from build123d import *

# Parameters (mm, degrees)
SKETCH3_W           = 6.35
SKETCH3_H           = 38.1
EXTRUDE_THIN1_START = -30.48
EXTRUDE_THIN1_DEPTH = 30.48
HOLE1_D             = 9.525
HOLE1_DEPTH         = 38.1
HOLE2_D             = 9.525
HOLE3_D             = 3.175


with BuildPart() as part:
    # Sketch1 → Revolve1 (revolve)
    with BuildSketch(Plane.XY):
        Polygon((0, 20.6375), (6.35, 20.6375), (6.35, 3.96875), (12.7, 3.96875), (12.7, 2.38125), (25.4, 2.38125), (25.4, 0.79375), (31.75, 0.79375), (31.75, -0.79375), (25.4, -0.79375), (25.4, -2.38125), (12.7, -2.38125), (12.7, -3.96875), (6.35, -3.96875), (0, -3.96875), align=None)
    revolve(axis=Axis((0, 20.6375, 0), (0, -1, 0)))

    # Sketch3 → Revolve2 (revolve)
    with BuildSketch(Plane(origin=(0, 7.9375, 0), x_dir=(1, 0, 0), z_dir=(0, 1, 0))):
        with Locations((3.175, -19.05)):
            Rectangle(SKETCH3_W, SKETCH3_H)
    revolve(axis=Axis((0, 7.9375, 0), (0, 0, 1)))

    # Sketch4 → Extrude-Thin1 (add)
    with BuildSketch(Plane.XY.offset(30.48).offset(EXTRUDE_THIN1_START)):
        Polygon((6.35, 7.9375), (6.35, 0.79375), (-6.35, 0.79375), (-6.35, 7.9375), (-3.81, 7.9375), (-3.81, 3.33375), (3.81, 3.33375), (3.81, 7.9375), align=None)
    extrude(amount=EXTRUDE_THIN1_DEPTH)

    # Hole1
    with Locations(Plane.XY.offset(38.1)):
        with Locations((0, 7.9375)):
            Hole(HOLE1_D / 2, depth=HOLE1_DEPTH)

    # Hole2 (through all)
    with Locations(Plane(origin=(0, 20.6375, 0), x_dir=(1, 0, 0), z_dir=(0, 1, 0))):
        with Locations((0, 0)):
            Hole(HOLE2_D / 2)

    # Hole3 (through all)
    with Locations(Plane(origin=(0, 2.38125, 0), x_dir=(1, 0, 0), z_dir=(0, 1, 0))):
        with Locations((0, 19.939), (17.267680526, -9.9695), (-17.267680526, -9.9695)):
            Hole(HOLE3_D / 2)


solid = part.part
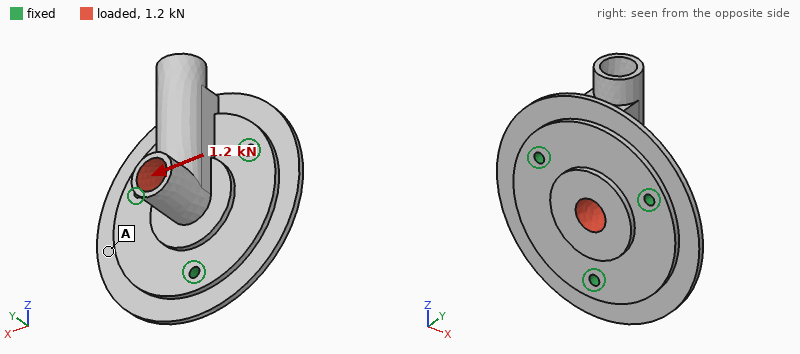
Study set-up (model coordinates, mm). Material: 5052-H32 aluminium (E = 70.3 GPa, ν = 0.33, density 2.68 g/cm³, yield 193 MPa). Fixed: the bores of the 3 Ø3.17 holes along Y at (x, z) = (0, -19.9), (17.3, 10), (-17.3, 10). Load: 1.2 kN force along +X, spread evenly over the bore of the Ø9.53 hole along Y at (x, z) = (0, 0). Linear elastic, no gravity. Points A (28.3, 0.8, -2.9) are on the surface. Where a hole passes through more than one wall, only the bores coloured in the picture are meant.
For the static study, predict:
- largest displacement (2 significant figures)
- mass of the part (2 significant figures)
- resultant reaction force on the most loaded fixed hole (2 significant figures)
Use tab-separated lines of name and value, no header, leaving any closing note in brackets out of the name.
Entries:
largest displacement	28 µm
mass of the part	41 g
resultant reaction force on the most loaded fixed hole	530 N
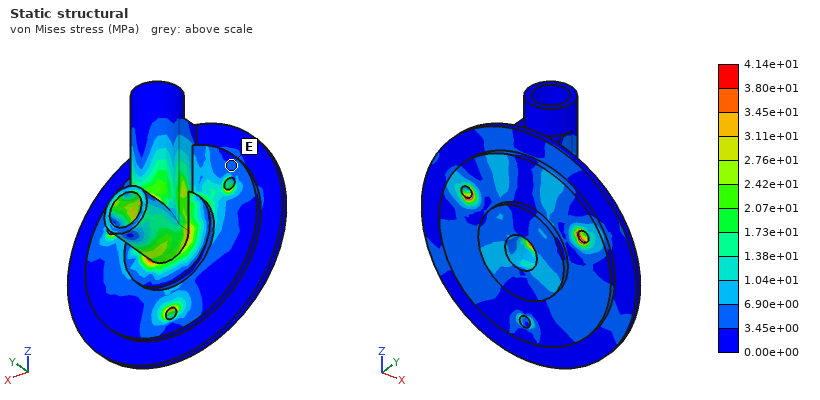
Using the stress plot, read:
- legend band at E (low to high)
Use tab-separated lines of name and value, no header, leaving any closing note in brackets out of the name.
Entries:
legend band at E	3.45e+00 to 6.90e+00 MPa
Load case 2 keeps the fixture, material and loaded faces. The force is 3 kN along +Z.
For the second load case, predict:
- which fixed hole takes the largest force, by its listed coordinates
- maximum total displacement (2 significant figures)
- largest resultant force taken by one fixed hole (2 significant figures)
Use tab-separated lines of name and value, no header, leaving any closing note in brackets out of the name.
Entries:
which fixed hole takes the largest force, by its listed coordinates	(0, -19.9)
maximum total displacement	63 µm
largest resultant force taken by one fixed hole	1.3 kN
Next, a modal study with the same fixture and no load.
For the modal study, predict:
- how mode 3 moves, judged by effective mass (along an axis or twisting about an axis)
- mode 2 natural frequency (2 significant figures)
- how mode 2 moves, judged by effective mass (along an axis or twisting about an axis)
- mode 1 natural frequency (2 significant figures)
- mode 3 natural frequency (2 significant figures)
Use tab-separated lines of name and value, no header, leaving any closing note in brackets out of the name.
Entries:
how mode 3 moves, judged by effective mass	along Y
mode 2 natural frequency	10 kHz
how mode 2 moves, judged by effective mass	twisting about Z
mode 1 natural frequency	7600 Hz
mode 3 natural frequency	11 kHz
